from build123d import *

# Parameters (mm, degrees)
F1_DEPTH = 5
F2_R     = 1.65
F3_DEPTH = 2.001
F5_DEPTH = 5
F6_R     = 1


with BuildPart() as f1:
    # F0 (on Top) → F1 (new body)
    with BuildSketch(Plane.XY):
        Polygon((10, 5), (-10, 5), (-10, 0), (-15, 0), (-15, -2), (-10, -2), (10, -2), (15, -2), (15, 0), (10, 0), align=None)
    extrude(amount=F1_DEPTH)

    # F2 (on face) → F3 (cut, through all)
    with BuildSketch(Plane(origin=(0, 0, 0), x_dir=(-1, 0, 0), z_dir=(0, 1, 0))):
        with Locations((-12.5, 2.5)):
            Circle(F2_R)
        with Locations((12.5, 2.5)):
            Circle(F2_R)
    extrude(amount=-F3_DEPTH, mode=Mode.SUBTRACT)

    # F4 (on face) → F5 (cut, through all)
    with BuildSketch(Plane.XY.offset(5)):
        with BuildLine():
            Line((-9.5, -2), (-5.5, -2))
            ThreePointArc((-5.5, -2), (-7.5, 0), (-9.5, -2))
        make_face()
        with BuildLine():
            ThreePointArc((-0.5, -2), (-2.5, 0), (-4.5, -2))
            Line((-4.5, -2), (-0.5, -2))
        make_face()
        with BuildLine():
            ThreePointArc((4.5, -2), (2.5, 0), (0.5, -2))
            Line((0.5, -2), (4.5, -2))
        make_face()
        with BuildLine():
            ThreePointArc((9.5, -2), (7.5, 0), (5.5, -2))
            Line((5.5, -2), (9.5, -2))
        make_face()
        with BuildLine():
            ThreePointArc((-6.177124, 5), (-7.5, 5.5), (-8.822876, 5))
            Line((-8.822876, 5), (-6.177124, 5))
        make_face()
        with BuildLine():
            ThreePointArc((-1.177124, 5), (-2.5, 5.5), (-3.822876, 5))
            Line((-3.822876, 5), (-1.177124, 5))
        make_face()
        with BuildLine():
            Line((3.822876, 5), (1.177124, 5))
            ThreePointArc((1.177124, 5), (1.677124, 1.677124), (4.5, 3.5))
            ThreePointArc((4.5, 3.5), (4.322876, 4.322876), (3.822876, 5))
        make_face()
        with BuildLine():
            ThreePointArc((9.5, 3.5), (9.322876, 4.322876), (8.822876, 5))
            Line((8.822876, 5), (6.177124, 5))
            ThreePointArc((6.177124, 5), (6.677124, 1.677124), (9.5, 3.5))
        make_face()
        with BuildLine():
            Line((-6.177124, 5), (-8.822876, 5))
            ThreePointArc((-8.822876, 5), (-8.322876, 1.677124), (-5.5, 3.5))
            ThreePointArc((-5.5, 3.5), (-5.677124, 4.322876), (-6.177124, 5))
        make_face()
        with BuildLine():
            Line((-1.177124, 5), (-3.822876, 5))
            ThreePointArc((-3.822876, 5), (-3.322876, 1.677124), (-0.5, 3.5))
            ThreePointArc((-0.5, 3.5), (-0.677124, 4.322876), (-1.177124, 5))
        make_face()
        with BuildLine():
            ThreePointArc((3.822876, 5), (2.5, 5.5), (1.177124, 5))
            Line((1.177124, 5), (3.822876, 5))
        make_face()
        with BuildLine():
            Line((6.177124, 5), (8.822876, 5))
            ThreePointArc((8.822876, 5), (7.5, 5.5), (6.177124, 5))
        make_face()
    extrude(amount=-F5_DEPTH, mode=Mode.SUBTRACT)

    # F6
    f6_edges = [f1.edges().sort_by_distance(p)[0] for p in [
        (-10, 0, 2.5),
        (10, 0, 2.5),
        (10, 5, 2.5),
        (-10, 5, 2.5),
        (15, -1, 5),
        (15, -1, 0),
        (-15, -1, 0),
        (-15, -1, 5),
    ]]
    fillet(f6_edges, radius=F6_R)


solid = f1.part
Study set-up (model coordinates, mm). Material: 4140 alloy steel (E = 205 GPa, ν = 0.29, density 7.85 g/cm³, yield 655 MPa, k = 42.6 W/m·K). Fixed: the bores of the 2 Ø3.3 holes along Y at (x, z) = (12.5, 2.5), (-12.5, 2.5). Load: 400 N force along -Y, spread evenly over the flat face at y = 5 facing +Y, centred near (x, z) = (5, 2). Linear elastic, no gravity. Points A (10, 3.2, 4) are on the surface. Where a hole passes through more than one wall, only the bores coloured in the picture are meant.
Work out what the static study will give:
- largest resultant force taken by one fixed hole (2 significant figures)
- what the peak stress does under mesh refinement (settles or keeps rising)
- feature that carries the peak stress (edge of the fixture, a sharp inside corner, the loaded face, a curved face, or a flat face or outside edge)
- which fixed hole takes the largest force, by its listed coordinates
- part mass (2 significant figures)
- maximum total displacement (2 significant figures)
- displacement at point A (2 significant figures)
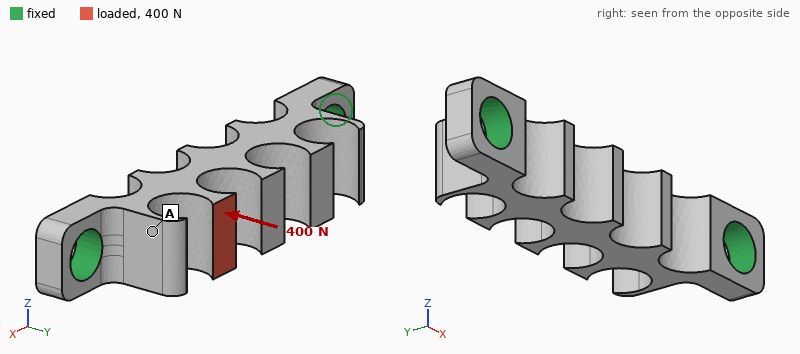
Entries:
450 N
keeps rising
edge of the fixture
(12.5, 2.5)
3.2 g
26 µm
9.3 µm
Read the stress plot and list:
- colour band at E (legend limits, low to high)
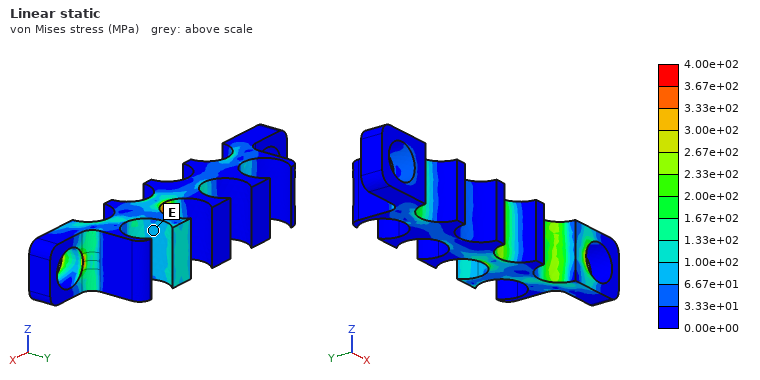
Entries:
6.67e+01 to 1.00e+02 MPa
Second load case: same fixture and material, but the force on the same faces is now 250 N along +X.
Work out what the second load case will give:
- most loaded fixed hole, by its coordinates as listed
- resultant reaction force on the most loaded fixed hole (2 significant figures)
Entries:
(-12.5, 2.5)
210 N
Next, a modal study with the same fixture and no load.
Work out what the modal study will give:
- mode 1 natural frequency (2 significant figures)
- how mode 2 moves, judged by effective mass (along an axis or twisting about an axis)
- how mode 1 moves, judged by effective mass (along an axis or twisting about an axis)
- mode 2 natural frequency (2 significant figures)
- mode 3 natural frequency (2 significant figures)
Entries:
16 kHz
along Z
along Y
24 kHz
30 kHz
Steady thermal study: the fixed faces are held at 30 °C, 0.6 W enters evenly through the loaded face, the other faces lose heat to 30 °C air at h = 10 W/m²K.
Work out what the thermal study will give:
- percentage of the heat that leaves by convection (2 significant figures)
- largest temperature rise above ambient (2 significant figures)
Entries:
3.7 %
15 K
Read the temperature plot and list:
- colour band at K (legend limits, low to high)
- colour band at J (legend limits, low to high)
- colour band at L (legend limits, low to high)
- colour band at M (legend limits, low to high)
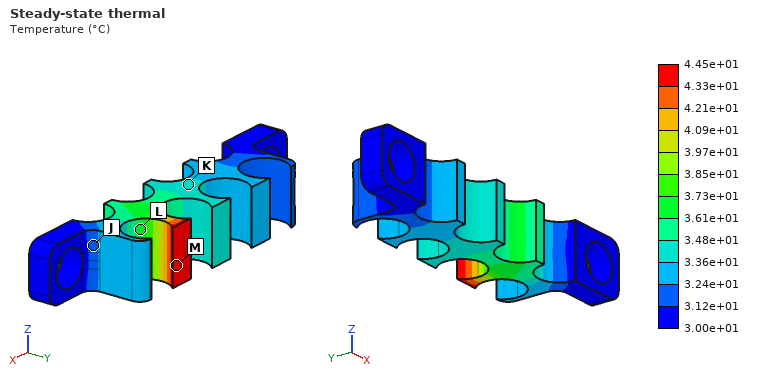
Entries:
3.36e+01 to 3.48e+01 °C
3.12e+01 to 3.24e+01 °C
3.61e+01 to 3.73e+01 °C
4.33e+01 to 4.45e+01 °C
